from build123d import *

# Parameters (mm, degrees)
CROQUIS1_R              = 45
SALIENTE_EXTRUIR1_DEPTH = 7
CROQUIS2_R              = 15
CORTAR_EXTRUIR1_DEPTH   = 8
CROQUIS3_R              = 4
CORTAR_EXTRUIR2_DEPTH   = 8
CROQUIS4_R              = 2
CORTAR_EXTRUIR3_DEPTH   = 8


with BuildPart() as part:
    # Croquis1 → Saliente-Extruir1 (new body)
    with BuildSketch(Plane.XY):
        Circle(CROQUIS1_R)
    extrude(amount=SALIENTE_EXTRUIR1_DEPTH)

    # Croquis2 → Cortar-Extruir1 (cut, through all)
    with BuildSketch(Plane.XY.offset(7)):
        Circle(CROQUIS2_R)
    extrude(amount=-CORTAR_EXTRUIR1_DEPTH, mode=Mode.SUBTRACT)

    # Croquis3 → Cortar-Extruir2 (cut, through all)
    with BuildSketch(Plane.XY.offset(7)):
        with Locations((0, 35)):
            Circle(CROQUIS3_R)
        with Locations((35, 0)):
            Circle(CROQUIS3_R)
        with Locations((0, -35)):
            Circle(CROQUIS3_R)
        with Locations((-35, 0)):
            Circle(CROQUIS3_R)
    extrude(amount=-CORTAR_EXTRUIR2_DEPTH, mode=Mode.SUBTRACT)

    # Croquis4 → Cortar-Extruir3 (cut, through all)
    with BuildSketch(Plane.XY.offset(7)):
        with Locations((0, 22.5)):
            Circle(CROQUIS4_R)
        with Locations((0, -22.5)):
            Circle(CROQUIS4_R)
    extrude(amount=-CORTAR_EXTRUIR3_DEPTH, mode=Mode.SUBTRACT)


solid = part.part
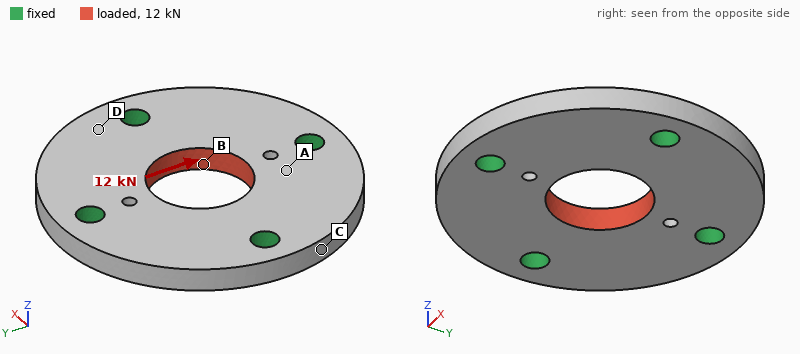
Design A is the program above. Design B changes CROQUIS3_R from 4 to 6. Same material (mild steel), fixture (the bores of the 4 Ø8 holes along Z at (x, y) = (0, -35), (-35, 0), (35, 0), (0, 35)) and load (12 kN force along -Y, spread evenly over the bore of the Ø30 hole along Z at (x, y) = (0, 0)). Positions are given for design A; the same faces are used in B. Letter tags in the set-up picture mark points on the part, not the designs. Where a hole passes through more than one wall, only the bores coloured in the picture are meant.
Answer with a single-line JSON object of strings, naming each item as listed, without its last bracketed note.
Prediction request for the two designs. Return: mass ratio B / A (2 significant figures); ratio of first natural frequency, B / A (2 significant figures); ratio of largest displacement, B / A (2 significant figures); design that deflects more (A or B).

{"mass ratio B / A": "0.95", "ratio of first natural frequency, B / A": "1.2", "ratio of largest displacement, B / A": "0.86", "design that deflects more": "A"}
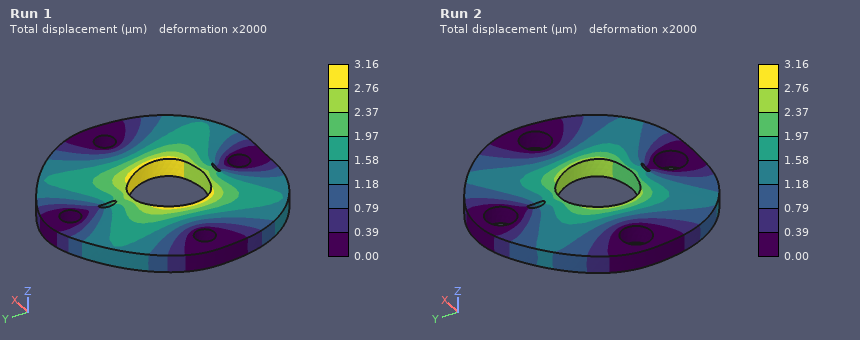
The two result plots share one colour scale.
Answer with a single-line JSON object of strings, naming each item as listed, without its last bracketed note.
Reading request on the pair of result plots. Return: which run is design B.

{"which run is design B": "Run 2"}
